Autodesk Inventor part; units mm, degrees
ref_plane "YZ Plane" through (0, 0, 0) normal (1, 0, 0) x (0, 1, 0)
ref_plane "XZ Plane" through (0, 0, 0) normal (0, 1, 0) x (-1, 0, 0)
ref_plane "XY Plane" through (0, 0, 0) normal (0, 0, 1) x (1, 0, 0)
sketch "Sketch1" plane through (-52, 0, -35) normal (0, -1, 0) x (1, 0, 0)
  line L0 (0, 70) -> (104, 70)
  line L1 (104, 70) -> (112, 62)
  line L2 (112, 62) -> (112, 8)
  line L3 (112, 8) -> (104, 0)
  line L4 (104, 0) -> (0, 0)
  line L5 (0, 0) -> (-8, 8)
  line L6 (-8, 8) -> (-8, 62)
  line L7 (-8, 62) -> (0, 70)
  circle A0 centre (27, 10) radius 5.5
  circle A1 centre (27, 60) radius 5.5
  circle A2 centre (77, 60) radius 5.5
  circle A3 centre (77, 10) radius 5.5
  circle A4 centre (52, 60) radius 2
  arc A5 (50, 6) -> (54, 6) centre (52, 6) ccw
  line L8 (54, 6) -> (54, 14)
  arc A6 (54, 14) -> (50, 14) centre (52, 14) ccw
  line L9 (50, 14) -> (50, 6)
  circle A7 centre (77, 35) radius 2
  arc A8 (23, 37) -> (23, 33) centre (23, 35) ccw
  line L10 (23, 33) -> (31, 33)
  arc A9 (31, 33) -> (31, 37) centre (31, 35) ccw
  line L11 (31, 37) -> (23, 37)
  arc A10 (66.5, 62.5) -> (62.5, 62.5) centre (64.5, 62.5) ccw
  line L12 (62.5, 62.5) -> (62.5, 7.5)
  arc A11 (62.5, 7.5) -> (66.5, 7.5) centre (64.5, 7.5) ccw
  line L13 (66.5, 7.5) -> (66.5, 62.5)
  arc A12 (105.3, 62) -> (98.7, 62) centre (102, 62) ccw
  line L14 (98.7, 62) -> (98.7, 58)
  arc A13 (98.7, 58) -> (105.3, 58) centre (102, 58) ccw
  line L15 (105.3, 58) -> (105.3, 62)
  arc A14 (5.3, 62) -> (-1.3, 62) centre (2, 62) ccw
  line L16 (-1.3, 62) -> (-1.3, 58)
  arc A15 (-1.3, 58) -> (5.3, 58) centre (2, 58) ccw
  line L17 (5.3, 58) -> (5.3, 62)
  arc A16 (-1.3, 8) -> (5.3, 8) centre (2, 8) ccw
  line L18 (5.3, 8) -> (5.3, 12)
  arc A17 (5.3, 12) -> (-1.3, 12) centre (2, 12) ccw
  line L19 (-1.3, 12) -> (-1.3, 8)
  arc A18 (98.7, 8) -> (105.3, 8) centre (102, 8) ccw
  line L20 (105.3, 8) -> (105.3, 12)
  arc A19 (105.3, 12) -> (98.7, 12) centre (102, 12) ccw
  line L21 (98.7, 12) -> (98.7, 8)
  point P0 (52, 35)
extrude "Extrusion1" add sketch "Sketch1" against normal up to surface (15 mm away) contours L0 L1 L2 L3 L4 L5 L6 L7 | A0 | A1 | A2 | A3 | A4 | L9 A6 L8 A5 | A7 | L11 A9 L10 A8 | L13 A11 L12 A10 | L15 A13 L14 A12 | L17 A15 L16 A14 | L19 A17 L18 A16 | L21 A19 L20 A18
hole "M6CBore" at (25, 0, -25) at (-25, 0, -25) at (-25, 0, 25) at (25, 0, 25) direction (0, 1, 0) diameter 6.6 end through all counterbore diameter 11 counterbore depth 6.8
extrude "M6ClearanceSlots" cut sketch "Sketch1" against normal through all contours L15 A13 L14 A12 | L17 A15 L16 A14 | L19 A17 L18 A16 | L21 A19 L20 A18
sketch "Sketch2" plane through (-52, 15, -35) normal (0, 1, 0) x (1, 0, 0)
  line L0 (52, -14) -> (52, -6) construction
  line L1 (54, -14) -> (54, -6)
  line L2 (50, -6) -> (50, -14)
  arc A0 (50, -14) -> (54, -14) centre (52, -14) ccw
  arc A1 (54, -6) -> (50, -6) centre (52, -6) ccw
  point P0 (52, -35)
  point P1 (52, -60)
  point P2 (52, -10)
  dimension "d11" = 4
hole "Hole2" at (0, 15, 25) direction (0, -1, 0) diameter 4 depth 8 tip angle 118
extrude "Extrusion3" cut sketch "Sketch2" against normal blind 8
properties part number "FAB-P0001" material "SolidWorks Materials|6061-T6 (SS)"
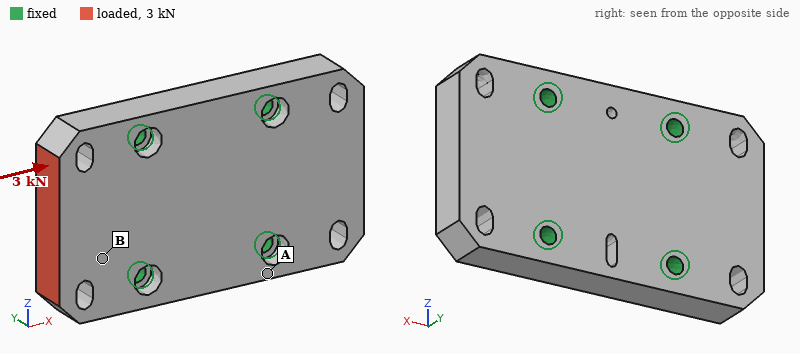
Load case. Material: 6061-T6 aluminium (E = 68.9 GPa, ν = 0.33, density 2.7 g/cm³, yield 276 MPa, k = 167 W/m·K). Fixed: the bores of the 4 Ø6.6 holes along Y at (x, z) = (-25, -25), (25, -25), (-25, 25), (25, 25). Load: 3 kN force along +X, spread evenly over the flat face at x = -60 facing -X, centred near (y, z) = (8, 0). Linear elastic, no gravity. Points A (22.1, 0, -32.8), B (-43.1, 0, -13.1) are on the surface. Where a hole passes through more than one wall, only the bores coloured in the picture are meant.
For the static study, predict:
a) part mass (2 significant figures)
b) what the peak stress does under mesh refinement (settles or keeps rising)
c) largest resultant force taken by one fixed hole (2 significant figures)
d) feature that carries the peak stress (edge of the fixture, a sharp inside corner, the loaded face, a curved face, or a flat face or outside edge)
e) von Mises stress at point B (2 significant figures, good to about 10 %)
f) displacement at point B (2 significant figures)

310 g
keeps rising
1.1 kN
edge of the fixture
4.0 MPa
2.9 µm
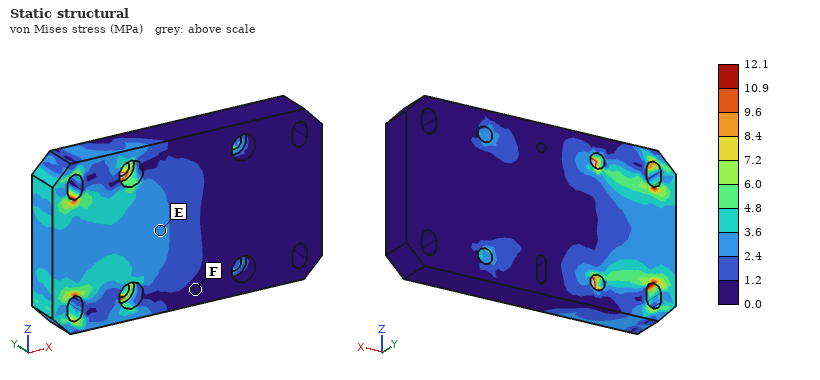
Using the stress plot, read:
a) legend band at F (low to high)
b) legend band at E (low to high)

0.0 to 1.2 MPa
2.4 to 3.6 MPa
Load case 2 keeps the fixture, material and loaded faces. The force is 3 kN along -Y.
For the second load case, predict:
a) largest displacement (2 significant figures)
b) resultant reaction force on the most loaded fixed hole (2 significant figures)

77 µm
2.6 kN
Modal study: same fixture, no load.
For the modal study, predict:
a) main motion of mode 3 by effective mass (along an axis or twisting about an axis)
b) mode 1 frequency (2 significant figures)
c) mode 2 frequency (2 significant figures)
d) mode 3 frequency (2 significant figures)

twisting about X
6400 Hz
6400 Hz
12 kHz
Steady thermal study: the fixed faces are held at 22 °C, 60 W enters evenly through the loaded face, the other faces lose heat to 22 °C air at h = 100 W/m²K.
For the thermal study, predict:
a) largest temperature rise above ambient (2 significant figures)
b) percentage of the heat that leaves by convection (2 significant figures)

17 K
12 %
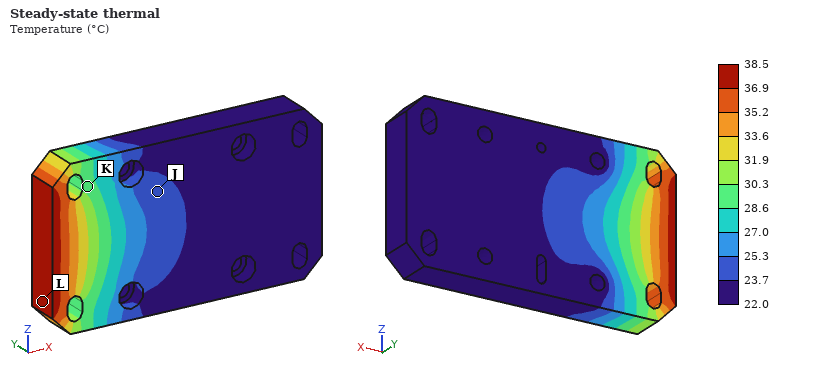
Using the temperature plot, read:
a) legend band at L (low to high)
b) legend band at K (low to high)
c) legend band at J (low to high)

36.9 to 38.5 °C
28.6 to 30.3 °C
23.7 to 25.3 °C
